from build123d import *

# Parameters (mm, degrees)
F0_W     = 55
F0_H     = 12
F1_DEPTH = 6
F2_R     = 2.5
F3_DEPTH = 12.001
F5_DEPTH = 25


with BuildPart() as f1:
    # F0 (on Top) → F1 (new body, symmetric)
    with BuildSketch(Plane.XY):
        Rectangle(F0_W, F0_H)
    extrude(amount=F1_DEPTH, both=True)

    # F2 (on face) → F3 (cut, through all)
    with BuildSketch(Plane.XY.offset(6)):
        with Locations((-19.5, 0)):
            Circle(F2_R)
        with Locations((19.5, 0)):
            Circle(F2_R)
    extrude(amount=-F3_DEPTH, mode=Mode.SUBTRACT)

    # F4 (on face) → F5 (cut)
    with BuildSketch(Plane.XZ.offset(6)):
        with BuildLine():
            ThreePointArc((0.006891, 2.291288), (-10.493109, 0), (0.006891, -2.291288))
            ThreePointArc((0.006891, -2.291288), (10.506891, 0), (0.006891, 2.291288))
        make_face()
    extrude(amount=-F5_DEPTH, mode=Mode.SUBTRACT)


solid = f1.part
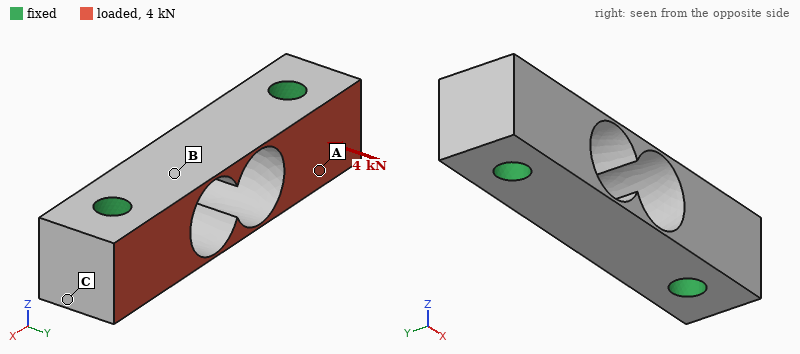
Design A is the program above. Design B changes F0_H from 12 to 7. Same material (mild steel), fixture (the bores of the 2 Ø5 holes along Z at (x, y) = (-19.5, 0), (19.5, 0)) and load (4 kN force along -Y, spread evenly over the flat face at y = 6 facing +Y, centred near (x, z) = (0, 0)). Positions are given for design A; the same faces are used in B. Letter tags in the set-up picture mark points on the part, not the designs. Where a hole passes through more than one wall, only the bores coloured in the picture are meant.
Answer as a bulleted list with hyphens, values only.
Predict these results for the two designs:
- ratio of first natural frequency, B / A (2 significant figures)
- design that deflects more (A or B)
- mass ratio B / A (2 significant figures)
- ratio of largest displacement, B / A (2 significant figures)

- 0.99
- B
- 0.55
- 2.7
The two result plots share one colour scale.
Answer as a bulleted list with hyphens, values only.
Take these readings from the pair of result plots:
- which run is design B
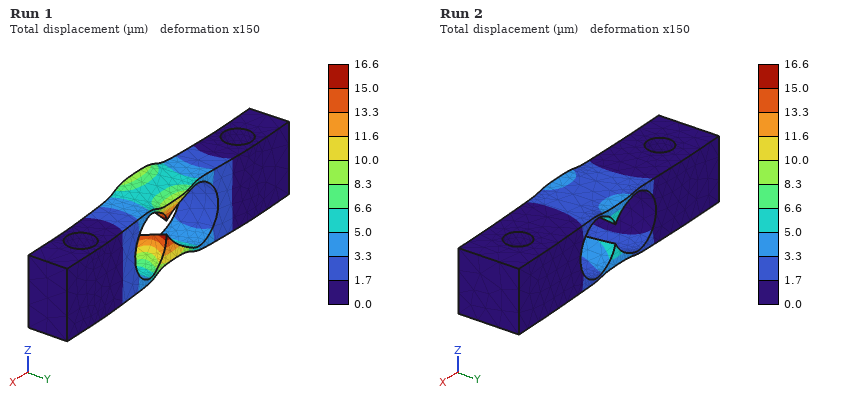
- Run 1
